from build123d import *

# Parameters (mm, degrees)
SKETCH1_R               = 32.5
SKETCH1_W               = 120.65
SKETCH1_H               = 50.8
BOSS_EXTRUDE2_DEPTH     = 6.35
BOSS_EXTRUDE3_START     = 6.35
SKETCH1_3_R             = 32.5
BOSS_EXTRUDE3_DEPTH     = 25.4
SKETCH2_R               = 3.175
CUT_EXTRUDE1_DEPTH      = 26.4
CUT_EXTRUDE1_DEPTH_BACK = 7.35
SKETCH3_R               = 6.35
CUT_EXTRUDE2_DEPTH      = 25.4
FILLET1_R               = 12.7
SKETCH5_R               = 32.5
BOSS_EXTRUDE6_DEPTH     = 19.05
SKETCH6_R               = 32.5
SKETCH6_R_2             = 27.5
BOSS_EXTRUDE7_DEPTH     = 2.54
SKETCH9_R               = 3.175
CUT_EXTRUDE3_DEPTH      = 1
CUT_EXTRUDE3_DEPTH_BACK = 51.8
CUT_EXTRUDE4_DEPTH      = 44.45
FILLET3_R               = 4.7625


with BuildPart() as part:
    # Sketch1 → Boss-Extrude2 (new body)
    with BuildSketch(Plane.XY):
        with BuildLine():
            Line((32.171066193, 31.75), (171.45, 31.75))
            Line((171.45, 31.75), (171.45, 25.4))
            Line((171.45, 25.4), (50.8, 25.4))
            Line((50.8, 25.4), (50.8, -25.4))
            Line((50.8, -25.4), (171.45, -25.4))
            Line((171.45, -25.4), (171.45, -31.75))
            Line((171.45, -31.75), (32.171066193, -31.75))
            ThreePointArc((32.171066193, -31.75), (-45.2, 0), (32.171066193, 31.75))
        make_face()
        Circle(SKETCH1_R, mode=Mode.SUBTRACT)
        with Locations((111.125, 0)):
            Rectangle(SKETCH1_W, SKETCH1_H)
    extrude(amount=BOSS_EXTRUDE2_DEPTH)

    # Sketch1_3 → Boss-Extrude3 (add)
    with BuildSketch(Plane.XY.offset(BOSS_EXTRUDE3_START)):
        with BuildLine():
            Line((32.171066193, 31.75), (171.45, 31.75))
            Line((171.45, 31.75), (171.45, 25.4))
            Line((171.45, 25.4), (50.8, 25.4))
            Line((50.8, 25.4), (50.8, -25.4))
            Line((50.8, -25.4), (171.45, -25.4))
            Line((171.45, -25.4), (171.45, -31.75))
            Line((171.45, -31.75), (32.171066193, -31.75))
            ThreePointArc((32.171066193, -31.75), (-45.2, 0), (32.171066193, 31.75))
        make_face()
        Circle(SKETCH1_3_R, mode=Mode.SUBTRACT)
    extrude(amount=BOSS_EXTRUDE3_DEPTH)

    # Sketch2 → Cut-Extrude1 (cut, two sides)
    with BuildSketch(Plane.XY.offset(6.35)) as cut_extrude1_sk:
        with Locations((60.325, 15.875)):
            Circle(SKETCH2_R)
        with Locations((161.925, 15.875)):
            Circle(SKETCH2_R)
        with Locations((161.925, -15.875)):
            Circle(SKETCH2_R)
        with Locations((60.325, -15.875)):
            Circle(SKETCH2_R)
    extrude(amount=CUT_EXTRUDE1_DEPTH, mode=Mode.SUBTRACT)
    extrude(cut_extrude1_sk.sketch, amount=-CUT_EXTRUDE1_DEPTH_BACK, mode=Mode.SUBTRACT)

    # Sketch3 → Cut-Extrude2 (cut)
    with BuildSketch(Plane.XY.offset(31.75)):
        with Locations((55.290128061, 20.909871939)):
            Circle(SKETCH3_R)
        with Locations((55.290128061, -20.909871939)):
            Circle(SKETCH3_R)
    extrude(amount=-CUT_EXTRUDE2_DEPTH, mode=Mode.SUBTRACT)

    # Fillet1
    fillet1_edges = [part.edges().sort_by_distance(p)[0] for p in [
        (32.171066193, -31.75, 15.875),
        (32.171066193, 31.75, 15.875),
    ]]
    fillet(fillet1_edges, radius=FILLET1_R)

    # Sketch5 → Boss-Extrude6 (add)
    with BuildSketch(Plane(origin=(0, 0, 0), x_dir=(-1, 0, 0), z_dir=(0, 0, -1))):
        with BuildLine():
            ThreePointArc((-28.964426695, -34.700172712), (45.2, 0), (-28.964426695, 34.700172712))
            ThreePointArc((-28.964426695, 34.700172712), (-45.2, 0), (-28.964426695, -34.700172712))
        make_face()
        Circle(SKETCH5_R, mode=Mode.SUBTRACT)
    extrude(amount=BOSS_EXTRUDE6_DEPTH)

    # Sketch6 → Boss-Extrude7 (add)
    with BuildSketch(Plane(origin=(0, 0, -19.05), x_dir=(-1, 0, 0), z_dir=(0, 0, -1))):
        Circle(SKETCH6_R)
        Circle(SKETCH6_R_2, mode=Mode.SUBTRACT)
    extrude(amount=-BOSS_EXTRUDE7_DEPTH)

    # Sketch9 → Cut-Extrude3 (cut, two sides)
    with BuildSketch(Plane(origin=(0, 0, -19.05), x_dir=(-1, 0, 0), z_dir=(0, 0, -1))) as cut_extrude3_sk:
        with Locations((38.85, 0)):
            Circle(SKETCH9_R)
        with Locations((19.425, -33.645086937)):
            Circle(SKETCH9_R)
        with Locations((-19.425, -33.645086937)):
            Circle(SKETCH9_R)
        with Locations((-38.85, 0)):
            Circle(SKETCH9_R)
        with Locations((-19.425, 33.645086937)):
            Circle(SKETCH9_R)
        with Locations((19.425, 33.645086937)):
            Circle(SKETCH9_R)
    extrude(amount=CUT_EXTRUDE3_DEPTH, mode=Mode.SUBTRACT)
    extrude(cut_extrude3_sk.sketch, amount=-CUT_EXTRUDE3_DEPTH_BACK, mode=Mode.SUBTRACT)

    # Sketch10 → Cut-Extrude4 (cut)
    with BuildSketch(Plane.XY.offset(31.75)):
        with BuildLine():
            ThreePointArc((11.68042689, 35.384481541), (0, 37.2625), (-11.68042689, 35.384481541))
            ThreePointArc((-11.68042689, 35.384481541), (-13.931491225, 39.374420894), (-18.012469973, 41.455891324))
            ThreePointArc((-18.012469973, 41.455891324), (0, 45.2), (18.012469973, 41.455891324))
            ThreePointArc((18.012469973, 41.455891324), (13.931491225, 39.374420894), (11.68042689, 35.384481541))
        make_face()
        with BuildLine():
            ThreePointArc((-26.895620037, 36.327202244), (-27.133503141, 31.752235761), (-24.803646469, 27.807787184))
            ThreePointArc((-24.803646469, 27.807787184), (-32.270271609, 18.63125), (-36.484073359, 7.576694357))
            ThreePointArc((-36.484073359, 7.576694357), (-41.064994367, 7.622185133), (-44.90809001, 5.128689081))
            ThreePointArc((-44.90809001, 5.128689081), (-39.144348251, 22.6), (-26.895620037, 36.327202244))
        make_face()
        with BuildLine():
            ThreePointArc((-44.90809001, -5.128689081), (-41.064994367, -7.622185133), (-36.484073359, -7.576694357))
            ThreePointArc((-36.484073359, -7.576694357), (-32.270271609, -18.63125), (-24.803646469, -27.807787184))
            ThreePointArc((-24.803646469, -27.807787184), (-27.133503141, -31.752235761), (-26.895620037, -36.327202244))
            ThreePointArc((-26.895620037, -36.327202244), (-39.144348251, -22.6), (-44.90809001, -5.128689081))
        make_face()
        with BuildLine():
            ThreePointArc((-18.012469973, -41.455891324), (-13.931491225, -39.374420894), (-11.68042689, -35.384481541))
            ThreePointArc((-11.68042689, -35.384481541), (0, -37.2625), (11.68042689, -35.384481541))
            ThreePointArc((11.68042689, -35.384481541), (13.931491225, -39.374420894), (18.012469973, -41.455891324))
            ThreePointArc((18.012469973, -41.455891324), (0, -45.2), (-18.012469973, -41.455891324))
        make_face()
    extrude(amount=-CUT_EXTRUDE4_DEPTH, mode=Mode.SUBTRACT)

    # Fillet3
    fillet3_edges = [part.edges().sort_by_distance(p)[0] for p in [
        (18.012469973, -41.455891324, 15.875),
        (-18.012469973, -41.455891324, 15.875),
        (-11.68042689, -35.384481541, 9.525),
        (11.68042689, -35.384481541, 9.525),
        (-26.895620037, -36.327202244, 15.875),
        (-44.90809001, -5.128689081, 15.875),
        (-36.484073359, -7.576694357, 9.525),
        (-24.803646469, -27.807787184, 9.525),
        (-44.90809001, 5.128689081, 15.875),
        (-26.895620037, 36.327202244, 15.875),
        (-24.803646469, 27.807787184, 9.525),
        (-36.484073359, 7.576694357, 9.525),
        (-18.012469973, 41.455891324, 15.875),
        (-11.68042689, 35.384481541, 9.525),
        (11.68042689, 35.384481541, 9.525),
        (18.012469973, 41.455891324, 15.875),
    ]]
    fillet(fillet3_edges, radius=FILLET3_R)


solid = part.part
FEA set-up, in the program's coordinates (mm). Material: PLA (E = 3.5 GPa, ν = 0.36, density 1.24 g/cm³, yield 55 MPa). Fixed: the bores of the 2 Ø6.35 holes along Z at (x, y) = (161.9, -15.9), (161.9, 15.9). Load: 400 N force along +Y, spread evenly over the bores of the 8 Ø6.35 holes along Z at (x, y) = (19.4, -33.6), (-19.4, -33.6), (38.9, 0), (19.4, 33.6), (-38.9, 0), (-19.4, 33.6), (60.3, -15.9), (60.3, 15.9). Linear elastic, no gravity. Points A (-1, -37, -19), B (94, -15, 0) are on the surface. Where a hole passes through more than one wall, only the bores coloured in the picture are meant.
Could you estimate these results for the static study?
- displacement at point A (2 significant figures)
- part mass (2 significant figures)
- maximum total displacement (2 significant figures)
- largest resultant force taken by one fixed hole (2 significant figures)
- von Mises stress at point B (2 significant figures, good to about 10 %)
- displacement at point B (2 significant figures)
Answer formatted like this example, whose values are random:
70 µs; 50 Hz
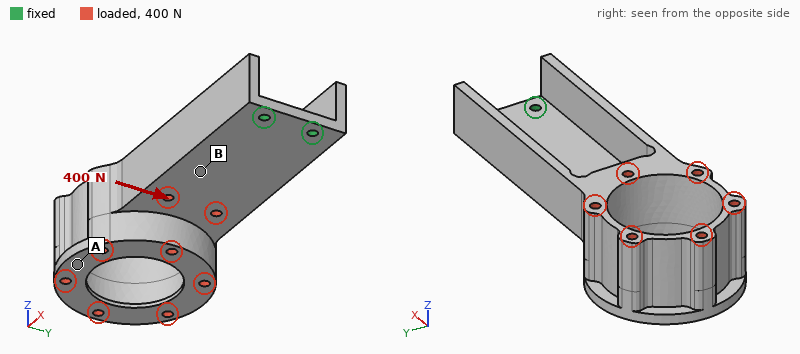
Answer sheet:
1.4 mm; 270 g; 1.9 mm; 1.8 kN; 3.0 MPa; 0.45 mm
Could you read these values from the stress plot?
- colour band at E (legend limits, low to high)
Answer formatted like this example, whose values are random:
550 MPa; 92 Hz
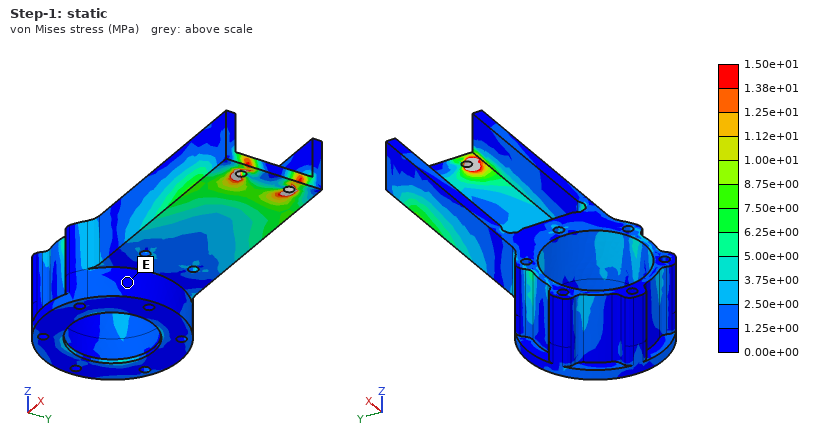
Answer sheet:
0.00e+00 to 1.25e+00 MPa
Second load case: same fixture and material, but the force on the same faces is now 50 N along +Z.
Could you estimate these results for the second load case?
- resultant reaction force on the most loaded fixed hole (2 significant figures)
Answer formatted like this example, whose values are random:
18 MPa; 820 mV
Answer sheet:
47 N
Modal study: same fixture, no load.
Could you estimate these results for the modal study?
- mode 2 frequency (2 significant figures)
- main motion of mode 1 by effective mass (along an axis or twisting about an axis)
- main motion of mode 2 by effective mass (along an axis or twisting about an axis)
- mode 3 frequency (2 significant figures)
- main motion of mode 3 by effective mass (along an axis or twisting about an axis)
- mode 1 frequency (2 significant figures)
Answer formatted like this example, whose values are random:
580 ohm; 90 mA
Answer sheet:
190 Hz; along Z; twisting about X; 220 Hz; along Y; 61 Hz
